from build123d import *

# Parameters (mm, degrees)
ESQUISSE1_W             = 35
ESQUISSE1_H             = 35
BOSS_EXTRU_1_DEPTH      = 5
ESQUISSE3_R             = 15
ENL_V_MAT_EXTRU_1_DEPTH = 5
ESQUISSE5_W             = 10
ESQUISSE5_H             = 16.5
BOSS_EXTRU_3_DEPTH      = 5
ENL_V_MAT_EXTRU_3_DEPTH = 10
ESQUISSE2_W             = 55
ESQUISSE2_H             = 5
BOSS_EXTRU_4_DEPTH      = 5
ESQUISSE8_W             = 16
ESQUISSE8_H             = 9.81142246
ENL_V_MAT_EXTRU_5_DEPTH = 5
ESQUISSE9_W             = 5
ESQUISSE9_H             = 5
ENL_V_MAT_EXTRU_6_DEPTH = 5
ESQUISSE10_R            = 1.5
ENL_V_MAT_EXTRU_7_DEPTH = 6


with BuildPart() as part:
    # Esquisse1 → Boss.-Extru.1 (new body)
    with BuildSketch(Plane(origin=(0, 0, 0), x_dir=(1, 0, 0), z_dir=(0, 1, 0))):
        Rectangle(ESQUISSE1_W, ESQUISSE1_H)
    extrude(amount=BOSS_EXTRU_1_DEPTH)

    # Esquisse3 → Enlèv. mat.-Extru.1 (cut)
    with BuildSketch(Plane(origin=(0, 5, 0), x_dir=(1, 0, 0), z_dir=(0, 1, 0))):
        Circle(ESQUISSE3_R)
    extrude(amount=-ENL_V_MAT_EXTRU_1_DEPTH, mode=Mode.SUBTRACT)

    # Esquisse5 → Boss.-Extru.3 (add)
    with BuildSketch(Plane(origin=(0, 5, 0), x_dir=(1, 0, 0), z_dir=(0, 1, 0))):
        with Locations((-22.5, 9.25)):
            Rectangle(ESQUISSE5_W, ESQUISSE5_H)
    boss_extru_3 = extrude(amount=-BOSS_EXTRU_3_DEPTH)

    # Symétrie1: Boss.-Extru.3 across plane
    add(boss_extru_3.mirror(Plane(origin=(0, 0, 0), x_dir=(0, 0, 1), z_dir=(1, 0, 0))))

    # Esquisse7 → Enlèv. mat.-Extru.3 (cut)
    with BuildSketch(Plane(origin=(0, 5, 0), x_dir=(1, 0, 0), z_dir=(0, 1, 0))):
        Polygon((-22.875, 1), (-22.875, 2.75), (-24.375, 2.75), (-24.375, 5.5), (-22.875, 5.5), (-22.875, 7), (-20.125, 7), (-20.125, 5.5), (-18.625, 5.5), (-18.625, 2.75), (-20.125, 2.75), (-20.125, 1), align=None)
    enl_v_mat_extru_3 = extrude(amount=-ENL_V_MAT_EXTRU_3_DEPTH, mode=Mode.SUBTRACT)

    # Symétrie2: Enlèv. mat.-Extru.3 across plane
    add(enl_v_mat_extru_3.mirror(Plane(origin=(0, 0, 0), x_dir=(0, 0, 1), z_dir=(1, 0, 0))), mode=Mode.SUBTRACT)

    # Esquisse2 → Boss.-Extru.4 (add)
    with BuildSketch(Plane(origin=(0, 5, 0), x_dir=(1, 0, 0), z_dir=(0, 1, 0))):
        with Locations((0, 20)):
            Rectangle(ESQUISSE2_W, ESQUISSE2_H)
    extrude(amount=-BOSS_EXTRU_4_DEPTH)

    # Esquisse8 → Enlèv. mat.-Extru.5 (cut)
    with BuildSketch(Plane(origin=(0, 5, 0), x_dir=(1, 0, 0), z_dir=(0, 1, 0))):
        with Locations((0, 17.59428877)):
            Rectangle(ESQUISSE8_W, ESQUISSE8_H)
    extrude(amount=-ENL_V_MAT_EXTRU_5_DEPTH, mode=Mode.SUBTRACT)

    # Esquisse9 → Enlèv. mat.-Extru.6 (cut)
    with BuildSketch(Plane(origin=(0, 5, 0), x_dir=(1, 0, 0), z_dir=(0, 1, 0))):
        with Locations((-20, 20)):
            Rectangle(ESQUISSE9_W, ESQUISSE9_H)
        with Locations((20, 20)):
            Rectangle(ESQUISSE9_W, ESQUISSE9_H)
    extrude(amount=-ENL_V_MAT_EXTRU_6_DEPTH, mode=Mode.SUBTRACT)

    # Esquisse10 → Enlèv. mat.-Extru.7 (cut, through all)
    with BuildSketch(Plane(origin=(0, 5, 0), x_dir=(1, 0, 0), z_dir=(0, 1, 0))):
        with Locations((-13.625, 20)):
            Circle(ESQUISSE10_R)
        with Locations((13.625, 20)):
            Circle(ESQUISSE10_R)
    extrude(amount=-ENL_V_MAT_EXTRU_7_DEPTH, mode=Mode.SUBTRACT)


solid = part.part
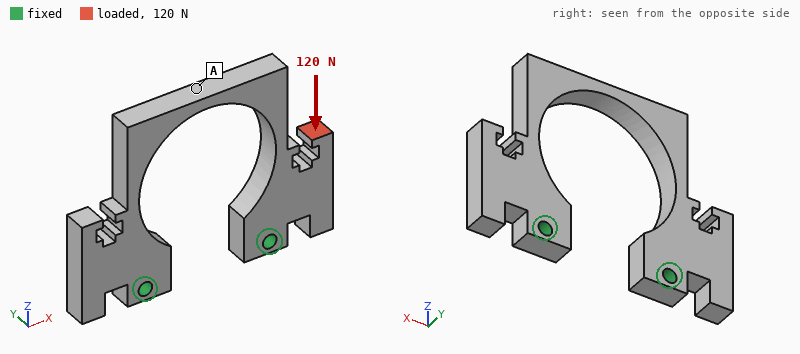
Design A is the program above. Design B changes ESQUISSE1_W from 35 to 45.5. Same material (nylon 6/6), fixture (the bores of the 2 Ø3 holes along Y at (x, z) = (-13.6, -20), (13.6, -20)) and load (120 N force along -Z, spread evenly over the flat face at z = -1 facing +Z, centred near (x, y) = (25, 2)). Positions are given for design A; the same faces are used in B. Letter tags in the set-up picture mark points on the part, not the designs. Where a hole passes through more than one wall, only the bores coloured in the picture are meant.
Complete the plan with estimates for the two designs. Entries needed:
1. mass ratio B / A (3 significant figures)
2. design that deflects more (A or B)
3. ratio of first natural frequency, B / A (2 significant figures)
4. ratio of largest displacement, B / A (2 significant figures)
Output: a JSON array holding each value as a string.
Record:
["1.22", "A", "0.87", "0.90"]
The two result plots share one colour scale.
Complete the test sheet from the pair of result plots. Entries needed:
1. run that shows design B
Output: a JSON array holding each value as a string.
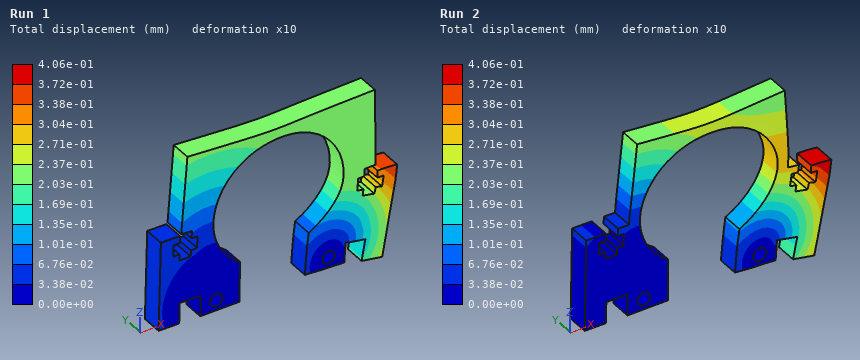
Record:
["Run 1"]
